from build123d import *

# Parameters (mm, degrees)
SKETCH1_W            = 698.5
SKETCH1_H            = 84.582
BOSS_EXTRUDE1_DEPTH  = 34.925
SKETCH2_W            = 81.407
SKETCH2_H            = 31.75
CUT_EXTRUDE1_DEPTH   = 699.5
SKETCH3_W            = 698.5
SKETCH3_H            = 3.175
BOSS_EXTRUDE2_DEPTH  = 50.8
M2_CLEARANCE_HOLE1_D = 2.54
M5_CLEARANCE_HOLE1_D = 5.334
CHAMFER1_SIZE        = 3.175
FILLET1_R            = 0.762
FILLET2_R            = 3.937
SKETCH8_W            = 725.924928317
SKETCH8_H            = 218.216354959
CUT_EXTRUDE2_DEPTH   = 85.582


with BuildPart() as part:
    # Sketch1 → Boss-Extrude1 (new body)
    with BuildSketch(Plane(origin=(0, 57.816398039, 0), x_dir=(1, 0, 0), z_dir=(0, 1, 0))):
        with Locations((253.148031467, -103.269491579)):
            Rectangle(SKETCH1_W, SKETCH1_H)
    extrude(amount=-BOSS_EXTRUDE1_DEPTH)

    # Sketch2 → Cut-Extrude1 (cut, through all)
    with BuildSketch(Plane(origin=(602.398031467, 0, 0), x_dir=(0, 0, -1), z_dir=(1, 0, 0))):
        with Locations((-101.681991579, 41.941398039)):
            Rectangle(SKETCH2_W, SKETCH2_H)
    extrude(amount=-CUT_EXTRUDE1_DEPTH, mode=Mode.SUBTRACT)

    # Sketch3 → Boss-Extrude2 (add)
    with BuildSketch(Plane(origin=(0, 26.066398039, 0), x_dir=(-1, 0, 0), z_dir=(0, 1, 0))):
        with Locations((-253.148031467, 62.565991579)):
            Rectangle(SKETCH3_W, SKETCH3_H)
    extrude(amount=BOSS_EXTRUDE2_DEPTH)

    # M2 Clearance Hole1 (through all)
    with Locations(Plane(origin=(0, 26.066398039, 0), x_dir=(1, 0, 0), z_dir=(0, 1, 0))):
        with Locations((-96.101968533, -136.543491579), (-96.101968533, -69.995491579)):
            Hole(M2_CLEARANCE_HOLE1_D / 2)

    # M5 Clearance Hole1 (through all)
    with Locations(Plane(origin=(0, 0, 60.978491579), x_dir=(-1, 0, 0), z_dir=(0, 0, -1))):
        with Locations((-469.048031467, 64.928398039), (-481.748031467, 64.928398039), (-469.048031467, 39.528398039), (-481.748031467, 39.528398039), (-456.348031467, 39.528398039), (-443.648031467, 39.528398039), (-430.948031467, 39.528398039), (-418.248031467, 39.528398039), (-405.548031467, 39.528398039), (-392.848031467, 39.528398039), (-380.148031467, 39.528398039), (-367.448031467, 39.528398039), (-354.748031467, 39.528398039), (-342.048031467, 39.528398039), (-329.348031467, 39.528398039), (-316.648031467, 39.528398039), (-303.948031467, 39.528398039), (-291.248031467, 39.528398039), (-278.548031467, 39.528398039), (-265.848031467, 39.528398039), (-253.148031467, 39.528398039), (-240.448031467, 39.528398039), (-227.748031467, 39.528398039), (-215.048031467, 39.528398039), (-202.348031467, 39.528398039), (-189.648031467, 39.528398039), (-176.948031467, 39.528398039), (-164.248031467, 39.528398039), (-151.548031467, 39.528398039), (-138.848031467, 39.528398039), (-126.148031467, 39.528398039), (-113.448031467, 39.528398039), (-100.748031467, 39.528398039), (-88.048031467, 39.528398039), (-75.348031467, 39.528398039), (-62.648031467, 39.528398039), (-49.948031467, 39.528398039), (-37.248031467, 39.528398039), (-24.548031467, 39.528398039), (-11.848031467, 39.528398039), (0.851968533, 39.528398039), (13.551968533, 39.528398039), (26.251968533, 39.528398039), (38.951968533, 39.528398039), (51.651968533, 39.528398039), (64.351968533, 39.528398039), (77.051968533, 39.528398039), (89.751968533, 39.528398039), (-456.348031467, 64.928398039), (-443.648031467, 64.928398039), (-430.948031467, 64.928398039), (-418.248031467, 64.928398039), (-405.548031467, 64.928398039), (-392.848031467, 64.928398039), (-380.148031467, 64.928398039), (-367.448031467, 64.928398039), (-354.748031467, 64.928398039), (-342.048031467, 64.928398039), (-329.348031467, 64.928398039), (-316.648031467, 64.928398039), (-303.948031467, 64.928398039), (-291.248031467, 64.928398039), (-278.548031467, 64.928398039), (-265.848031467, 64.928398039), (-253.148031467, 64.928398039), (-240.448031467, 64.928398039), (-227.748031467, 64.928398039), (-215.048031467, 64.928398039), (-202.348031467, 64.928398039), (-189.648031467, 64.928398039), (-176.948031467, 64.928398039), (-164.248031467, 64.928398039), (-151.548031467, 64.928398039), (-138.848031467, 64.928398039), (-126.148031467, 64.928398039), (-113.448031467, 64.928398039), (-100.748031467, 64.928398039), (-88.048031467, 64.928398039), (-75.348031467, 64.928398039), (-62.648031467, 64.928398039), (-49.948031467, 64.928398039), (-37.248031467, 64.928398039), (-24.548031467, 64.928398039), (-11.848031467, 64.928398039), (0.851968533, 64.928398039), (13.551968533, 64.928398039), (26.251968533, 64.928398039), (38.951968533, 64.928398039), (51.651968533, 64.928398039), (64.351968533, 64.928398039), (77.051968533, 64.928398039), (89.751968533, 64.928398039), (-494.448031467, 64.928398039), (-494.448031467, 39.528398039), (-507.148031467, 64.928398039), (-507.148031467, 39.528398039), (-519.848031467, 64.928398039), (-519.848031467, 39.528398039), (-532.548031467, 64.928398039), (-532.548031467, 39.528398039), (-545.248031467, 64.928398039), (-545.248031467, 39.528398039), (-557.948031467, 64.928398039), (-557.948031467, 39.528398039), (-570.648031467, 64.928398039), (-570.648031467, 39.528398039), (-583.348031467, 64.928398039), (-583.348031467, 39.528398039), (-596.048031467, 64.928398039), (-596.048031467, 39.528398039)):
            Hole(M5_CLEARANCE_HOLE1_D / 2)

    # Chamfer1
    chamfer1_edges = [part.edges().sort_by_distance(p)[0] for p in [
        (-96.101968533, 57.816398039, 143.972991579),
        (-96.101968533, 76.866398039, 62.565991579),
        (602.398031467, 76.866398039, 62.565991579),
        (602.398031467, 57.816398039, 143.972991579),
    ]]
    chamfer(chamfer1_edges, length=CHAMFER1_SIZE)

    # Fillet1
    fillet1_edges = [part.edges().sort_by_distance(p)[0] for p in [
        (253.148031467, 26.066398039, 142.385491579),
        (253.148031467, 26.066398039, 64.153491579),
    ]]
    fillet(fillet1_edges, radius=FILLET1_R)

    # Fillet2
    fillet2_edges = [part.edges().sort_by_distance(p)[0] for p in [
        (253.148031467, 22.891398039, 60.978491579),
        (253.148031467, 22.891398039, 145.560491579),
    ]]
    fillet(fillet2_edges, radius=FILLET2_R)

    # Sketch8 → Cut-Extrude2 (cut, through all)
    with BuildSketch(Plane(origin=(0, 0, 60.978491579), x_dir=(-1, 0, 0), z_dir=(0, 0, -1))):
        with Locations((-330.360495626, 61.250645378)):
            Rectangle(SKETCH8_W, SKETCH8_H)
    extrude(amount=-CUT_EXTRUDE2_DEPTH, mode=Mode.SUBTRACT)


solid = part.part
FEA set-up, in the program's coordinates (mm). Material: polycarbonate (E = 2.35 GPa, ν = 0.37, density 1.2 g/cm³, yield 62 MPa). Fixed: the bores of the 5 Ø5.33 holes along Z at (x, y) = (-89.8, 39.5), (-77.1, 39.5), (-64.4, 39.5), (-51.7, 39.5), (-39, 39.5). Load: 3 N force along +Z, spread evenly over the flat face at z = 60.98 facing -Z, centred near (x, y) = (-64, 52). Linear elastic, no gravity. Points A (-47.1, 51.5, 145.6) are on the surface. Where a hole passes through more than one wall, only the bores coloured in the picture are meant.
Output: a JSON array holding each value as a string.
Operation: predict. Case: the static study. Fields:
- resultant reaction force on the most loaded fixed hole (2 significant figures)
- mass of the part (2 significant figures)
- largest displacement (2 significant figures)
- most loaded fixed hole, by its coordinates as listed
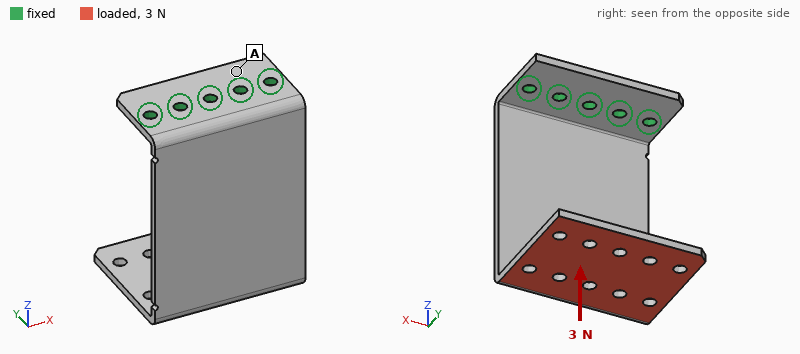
["1.0 N", "39 g", "1.3 mm", "(-64.4, 39.5)"]
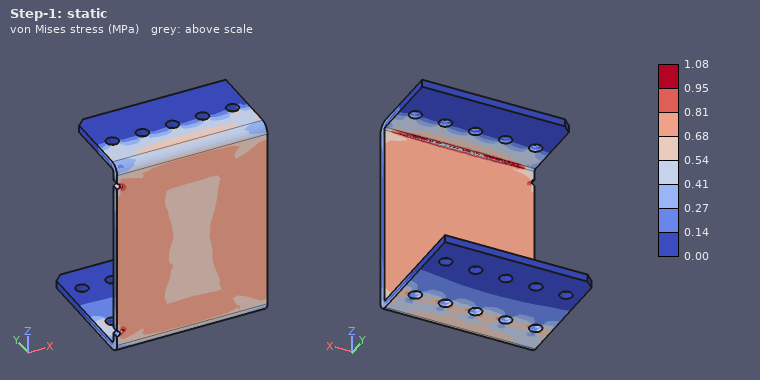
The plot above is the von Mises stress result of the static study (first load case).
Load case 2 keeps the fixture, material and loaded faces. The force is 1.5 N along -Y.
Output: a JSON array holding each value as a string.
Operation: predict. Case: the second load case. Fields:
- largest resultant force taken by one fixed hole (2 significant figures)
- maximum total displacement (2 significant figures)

["0.86 N", "1.2 mm"]
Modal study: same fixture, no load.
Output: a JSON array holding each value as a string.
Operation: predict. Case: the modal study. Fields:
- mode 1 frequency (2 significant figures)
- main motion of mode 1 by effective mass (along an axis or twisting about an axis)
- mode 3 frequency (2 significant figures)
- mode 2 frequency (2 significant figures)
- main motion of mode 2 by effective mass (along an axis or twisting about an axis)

["46 Hz", "along Y", "160 Hz", "100 Hz", "along X"]
